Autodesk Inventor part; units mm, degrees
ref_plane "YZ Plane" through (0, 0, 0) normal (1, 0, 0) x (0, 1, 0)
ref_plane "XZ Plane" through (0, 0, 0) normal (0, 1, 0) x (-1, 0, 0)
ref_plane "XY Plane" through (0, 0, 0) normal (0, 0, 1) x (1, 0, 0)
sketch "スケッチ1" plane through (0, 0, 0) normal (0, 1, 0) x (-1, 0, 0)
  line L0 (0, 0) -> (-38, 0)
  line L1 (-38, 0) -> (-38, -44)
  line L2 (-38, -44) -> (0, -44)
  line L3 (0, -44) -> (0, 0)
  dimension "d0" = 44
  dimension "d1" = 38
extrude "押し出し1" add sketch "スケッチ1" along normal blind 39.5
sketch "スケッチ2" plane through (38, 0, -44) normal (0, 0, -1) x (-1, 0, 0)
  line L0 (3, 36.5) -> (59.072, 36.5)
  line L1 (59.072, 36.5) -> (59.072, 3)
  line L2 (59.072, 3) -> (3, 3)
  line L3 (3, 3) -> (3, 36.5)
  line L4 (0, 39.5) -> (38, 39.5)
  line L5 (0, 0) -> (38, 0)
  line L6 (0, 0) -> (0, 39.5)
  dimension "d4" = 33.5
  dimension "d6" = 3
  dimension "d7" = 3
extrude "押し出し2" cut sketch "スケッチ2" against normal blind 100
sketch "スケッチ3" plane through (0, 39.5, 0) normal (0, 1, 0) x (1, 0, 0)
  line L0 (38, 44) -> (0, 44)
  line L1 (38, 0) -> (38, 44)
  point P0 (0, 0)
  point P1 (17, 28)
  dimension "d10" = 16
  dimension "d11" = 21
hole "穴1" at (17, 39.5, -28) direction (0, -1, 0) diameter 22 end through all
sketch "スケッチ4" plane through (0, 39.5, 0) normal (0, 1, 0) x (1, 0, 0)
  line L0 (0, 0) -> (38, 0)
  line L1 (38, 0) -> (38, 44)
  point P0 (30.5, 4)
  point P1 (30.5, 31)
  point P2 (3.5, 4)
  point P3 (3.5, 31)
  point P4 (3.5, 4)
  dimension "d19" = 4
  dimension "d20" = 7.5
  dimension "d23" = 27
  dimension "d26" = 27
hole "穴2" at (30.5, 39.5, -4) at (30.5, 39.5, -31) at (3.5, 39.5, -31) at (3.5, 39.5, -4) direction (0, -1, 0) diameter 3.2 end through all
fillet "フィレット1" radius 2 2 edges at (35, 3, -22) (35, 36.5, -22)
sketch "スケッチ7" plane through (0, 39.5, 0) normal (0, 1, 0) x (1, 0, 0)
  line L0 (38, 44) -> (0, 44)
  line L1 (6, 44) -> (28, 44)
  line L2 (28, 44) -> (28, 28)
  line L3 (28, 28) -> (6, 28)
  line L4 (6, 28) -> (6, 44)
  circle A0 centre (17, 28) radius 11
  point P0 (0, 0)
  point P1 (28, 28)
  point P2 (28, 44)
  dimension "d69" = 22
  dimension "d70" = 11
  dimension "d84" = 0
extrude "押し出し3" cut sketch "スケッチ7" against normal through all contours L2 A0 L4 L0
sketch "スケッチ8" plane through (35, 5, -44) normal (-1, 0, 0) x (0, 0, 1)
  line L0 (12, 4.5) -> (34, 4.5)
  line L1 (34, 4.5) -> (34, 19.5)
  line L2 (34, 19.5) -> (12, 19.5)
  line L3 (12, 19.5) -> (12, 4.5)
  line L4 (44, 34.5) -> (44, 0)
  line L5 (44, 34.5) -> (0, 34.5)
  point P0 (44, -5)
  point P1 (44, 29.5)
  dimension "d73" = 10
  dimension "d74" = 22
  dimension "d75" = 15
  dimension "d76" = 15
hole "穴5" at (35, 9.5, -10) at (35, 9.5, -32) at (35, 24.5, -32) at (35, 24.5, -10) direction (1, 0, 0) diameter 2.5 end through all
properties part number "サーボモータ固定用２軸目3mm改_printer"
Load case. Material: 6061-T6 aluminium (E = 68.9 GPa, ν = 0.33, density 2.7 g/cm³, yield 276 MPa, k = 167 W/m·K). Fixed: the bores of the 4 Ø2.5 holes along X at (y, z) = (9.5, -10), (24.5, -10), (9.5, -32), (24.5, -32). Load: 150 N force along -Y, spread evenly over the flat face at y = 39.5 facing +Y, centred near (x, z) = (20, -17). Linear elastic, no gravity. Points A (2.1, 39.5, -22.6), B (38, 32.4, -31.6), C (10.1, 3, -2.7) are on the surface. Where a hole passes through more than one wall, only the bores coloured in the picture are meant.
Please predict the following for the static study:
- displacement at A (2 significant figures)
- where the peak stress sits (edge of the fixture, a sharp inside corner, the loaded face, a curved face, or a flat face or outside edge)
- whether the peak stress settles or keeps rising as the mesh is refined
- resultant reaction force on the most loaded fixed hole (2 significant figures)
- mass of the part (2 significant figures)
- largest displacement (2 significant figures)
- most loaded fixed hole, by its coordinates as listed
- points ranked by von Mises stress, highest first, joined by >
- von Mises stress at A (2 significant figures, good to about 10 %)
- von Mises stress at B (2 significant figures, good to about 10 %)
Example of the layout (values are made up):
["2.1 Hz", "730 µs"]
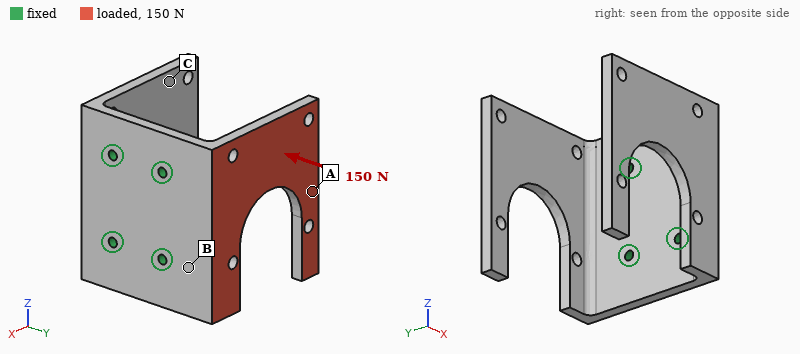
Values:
["0.42 mm", "edge of the fixture", "keeps rising", "85 N", "30 g", "0.54 mm", "(24.5, -10)", "B > A > C", "16 MPa", "26 MPa"]
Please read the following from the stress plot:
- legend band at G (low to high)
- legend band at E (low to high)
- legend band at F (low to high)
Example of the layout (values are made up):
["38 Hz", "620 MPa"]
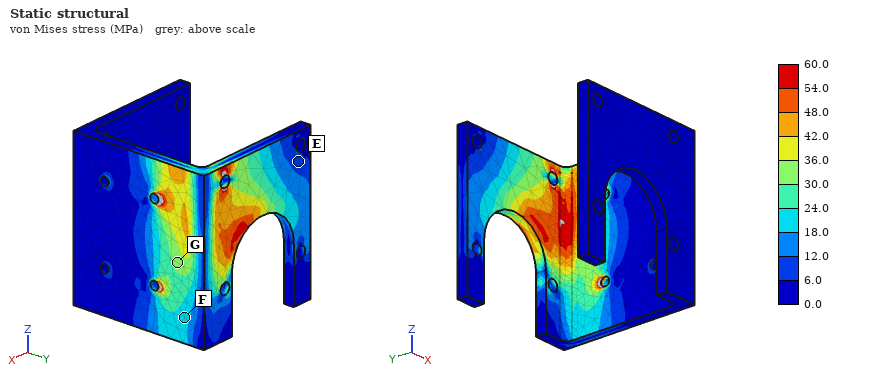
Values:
["30.0 to 36.0 MPa", "6.0 to 12.0 MPa", "18.0 to 24.0 MPa"]
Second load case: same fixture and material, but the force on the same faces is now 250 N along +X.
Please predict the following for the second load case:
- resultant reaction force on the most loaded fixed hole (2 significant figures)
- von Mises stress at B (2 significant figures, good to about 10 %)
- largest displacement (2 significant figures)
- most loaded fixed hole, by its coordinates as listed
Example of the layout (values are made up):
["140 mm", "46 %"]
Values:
["210 N", "23 MPa", "0.22 mm", "(24.5, -10)"]
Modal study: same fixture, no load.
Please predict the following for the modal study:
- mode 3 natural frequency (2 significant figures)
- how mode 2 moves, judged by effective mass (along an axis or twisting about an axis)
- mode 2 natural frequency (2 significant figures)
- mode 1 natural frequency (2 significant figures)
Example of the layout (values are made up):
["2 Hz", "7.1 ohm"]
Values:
["2300 Hz", "along Y", "1200 Hz", "1100 Hz"]
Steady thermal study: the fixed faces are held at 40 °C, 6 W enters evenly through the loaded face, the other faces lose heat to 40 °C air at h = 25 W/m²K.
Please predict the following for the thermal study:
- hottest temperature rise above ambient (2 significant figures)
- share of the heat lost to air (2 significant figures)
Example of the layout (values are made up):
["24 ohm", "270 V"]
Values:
["16 K", "8.2 %"]
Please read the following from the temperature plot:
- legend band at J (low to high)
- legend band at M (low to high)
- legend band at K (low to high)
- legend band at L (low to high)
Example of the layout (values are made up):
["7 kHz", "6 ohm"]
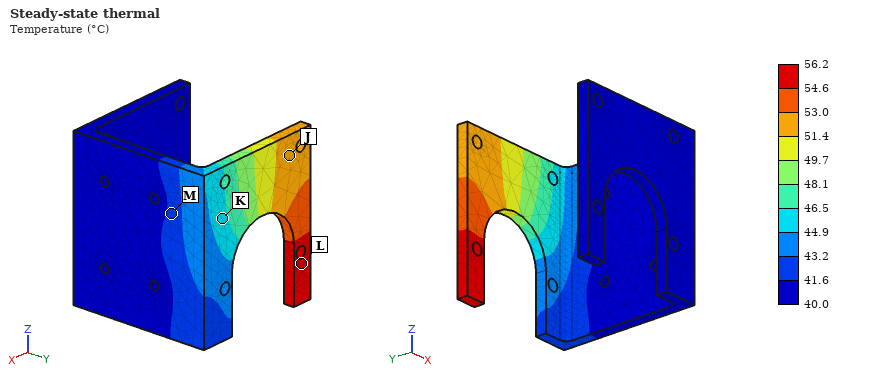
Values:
["51.4 to 53.0 °C", "41.6 to 43.2 °C", "44.9 to 46.5 °C", "54.6 to 56.2 °C"]
